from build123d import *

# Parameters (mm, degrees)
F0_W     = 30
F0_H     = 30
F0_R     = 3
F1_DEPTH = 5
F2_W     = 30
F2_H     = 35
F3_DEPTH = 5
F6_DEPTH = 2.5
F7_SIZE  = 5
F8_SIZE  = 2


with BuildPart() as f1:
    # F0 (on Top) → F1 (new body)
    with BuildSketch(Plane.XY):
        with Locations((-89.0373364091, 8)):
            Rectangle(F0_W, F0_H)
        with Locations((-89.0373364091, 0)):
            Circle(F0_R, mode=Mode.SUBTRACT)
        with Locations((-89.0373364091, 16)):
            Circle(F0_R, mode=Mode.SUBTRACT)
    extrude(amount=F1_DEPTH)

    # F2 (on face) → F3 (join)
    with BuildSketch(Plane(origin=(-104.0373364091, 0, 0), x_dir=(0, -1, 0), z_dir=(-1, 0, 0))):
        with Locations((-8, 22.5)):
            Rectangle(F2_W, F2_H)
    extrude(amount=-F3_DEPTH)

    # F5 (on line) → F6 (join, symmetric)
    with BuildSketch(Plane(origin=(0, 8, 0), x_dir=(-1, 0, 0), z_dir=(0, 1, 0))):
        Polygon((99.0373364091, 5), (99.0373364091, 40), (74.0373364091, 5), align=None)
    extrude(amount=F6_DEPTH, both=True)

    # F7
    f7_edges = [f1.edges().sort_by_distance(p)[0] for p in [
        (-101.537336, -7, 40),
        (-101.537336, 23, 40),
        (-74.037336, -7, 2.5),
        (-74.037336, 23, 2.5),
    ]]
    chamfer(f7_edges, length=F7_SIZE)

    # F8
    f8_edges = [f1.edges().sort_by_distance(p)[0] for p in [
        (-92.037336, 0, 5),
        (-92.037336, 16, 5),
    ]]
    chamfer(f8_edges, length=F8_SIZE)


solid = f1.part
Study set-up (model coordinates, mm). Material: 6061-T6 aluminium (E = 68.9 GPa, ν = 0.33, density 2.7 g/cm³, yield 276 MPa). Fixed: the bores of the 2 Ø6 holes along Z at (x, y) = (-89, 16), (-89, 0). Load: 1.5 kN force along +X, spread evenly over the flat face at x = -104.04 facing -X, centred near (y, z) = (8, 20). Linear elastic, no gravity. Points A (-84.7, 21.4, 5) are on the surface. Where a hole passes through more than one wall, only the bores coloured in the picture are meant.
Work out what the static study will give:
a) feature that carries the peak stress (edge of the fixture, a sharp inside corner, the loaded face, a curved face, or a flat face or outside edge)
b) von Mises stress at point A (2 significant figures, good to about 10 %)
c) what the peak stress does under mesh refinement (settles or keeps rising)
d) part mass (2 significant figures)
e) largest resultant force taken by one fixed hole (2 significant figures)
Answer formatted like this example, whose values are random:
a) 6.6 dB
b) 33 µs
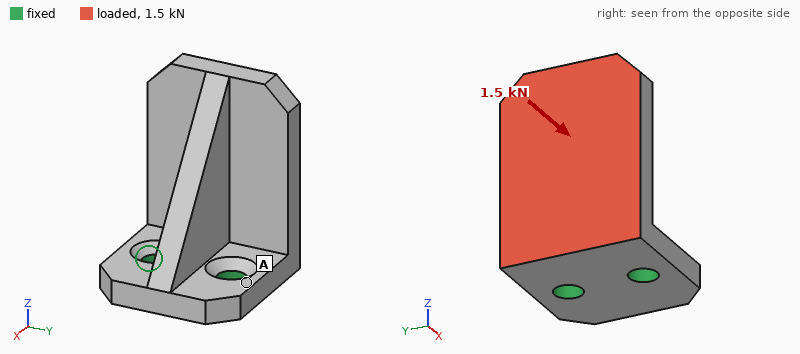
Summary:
a) edge of the fixture
b) 47 MPa
c) keeps rising
d) 31 g
e) 750 N
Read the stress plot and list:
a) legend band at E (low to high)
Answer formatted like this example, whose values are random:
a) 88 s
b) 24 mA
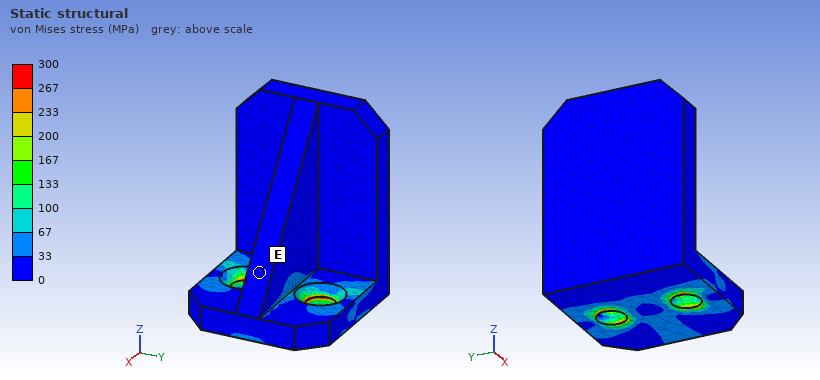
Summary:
a) 0 to 33 MPa
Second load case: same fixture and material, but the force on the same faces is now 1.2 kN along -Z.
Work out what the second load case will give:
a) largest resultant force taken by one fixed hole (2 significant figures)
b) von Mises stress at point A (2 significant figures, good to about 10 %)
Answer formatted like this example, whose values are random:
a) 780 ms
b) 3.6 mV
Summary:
a) 630 N
b) 23 MPa
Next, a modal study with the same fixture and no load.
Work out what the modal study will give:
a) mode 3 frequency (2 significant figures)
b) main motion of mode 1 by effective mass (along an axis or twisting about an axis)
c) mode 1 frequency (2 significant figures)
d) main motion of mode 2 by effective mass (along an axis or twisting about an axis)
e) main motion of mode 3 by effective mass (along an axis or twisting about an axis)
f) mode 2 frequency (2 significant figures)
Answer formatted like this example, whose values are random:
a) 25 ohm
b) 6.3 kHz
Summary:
a) 9600 Hz
b) along X
c) 3800 Hz
d) along Y
e) twisting about Z
f) 4900 Hz
